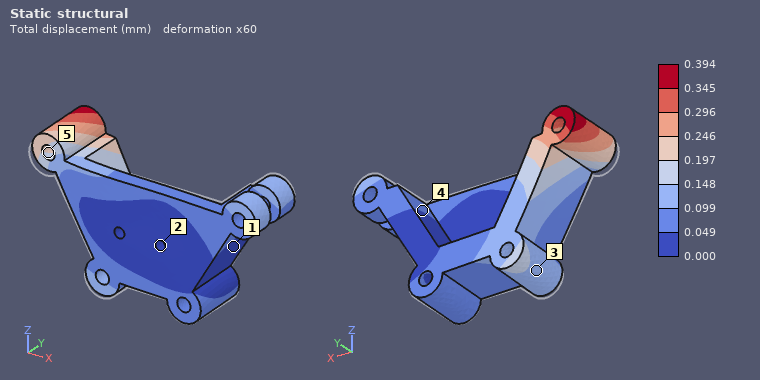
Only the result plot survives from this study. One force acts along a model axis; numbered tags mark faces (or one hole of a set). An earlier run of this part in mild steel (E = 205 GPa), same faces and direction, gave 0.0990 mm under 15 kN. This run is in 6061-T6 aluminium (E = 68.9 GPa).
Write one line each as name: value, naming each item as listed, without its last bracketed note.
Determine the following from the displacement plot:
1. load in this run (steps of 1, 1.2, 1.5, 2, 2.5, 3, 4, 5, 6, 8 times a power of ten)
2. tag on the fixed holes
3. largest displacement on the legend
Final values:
load in this run: 20 kN
tag on the fixed holes: 2
largest displacement on the legend: 0.394 mm
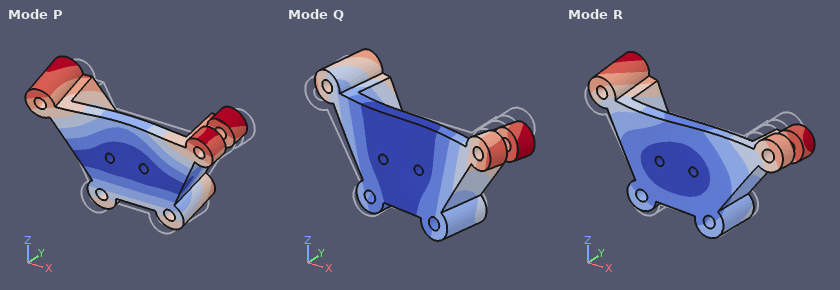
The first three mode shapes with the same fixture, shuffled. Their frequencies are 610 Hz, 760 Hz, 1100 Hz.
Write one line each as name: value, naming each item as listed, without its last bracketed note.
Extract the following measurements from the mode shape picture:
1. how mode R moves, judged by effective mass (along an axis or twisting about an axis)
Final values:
how mode R moves, judged by effective mass: twisting about Y
